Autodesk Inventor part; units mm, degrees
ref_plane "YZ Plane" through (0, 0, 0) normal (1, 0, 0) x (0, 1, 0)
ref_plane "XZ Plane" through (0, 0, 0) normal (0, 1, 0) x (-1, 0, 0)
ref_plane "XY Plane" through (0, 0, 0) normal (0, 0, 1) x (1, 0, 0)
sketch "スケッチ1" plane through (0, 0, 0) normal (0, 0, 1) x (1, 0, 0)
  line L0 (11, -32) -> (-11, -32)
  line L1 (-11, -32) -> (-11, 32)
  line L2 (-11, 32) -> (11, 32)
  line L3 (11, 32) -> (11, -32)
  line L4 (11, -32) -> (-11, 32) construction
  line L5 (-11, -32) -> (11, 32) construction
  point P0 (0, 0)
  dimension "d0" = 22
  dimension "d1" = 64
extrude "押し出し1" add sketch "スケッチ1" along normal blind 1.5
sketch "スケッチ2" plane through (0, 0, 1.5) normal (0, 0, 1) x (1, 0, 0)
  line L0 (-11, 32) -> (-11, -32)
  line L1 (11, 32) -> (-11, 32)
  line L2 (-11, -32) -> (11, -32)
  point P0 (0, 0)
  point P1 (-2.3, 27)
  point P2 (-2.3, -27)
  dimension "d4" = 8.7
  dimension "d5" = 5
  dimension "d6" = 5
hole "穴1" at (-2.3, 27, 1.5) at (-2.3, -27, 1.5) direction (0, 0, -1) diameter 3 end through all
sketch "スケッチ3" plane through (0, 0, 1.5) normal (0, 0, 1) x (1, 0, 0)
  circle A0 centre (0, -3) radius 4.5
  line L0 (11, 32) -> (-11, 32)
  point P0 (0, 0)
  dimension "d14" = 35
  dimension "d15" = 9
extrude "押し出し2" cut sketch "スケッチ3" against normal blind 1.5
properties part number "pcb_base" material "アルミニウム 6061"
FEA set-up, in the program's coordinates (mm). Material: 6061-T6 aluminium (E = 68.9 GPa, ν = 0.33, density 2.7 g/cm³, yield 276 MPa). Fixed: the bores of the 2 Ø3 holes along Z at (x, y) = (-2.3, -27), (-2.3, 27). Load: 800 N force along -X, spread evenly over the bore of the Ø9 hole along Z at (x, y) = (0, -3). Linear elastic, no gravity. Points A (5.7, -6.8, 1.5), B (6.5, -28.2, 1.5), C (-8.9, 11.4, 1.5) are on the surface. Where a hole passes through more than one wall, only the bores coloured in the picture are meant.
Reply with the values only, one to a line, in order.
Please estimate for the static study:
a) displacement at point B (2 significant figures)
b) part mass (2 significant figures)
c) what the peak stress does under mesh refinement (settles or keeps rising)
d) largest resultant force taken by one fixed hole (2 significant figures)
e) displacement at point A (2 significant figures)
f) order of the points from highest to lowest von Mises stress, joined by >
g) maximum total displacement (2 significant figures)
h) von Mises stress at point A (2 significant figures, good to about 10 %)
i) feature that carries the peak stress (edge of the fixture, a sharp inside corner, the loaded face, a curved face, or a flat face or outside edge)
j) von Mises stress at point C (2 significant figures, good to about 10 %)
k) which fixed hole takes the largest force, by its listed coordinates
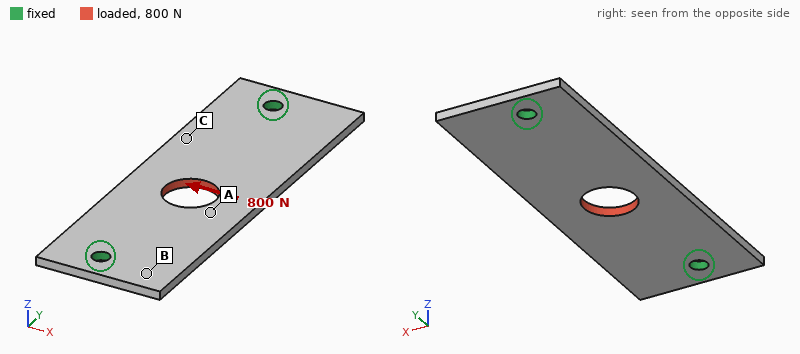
8.9 µm
5.4 g
keeps rising
470 N
32 µm
A > C > B
36 µm
45 MPa
edge of the fixture
24 MPa
(-2.3, -27)
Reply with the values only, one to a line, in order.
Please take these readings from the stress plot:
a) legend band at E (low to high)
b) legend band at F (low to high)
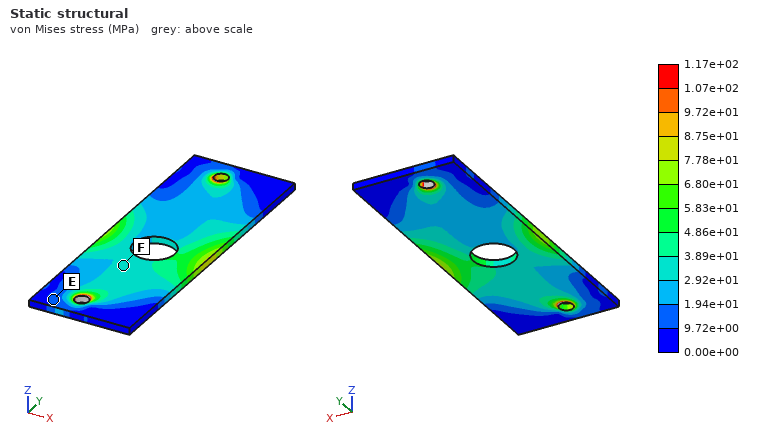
9.72e+00 to 1.94e+01 MPa
2.92e+01 to 3.89e+01 MPa
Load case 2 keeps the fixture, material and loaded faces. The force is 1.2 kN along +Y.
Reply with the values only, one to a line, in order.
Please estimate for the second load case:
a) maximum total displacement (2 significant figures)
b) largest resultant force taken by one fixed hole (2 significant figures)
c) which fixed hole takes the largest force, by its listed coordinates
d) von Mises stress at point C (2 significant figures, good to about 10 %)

11 µm
640 N
(-2.3, -27)
17 MPa
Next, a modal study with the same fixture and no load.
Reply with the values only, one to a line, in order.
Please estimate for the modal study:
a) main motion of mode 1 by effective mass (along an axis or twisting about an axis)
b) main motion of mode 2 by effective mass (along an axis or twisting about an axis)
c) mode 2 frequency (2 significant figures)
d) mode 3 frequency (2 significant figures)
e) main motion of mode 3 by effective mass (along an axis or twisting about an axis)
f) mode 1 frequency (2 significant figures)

along Z
twisting about Y
3800 Hz
6100 Hz
twisting about X
2500 Hz
